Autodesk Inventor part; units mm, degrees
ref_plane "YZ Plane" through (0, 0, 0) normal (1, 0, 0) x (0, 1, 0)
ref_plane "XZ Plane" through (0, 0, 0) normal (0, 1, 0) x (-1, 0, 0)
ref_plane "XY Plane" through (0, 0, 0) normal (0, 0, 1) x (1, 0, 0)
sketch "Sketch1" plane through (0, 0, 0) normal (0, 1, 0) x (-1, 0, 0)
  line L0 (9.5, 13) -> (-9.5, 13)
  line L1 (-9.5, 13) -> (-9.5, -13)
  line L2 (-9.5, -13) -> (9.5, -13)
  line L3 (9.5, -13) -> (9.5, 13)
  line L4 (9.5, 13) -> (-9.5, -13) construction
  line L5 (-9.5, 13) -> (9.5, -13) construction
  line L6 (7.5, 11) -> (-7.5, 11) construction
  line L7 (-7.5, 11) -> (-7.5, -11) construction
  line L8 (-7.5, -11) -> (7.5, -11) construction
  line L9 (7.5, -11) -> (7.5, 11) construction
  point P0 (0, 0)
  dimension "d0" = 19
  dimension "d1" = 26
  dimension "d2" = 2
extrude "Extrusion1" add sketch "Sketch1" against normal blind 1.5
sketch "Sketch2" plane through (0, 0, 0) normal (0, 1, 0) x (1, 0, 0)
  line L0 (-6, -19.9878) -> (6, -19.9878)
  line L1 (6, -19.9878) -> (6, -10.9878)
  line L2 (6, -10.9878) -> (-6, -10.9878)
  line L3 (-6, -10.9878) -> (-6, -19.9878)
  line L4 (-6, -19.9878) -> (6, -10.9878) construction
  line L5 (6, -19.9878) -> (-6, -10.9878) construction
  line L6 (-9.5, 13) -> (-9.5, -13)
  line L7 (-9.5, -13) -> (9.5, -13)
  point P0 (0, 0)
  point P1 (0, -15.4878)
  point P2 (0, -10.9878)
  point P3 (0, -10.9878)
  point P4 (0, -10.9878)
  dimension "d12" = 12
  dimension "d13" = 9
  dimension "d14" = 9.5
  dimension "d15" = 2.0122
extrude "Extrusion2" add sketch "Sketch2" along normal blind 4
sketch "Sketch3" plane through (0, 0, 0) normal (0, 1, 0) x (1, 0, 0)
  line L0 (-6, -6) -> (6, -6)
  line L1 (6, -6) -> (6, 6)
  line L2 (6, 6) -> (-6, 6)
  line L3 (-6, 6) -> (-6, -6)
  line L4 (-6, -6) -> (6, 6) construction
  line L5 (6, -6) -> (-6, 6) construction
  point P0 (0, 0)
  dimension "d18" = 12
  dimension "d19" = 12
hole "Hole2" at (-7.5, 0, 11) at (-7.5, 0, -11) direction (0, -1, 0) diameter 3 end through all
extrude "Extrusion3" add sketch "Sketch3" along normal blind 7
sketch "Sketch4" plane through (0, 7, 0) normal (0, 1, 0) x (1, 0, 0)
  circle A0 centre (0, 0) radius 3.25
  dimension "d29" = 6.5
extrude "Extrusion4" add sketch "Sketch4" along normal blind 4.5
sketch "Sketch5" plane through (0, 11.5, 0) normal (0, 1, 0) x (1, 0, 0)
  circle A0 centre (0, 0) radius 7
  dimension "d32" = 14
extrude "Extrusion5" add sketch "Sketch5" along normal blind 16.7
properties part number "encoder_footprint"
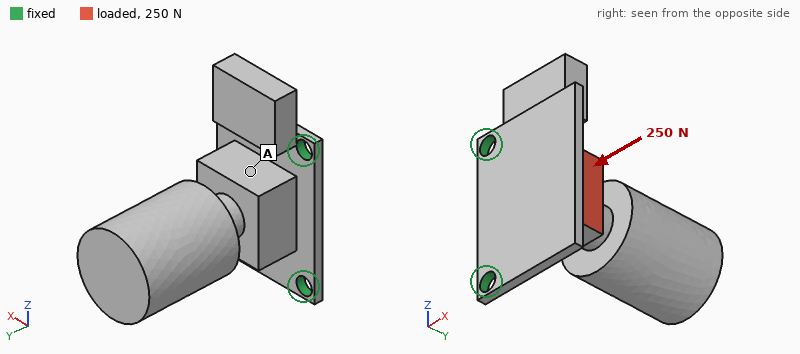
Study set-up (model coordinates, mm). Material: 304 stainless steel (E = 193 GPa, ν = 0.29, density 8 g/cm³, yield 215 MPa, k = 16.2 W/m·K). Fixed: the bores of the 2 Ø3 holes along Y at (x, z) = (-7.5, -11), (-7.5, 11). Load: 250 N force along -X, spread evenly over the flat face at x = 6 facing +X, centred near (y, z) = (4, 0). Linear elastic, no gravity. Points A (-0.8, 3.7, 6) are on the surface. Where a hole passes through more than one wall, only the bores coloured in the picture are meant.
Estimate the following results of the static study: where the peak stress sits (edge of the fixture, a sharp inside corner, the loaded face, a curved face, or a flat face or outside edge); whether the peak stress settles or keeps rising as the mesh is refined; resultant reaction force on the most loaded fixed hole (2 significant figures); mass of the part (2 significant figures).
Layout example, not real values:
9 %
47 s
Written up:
edge of the fixture
keeps rising
140 N
39 g
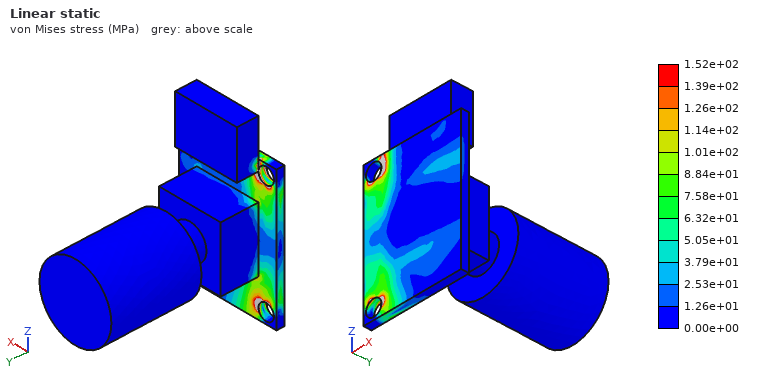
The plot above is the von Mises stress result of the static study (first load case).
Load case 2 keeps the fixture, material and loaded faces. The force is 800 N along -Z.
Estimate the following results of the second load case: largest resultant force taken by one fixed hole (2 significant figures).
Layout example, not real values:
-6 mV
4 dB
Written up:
660 N
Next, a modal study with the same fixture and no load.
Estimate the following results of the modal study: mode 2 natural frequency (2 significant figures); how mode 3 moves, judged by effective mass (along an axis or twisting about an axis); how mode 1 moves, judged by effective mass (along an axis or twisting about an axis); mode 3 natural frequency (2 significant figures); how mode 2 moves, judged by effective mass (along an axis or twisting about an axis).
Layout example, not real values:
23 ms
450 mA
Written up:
2300 Hz
along Y
along X
5300 Hz
along Z
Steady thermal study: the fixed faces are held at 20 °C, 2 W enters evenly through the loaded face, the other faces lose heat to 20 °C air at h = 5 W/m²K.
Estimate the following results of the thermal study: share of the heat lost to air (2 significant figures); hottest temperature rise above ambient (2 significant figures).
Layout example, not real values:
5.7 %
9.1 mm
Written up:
15 %
33 K
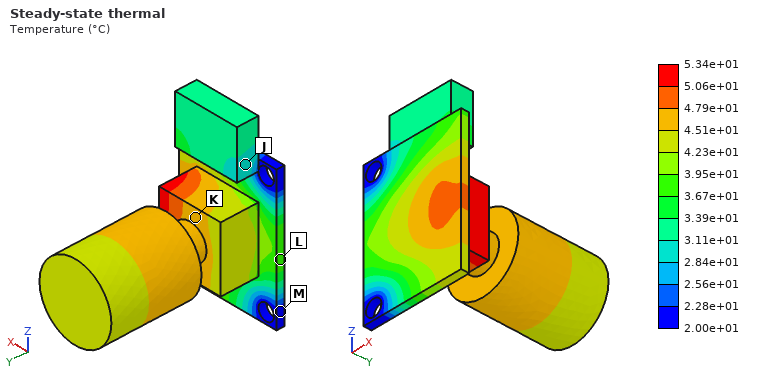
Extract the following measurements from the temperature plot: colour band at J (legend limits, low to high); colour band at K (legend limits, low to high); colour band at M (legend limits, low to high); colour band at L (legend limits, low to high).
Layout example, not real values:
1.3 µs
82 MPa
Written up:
2.84e+01 to 3.11e+01 °C
4.51e+01 to 4.79e+01 °C
2.00e+01 to 2.28e+01 °C
3.67e+01 to 3.95e+01 °C
